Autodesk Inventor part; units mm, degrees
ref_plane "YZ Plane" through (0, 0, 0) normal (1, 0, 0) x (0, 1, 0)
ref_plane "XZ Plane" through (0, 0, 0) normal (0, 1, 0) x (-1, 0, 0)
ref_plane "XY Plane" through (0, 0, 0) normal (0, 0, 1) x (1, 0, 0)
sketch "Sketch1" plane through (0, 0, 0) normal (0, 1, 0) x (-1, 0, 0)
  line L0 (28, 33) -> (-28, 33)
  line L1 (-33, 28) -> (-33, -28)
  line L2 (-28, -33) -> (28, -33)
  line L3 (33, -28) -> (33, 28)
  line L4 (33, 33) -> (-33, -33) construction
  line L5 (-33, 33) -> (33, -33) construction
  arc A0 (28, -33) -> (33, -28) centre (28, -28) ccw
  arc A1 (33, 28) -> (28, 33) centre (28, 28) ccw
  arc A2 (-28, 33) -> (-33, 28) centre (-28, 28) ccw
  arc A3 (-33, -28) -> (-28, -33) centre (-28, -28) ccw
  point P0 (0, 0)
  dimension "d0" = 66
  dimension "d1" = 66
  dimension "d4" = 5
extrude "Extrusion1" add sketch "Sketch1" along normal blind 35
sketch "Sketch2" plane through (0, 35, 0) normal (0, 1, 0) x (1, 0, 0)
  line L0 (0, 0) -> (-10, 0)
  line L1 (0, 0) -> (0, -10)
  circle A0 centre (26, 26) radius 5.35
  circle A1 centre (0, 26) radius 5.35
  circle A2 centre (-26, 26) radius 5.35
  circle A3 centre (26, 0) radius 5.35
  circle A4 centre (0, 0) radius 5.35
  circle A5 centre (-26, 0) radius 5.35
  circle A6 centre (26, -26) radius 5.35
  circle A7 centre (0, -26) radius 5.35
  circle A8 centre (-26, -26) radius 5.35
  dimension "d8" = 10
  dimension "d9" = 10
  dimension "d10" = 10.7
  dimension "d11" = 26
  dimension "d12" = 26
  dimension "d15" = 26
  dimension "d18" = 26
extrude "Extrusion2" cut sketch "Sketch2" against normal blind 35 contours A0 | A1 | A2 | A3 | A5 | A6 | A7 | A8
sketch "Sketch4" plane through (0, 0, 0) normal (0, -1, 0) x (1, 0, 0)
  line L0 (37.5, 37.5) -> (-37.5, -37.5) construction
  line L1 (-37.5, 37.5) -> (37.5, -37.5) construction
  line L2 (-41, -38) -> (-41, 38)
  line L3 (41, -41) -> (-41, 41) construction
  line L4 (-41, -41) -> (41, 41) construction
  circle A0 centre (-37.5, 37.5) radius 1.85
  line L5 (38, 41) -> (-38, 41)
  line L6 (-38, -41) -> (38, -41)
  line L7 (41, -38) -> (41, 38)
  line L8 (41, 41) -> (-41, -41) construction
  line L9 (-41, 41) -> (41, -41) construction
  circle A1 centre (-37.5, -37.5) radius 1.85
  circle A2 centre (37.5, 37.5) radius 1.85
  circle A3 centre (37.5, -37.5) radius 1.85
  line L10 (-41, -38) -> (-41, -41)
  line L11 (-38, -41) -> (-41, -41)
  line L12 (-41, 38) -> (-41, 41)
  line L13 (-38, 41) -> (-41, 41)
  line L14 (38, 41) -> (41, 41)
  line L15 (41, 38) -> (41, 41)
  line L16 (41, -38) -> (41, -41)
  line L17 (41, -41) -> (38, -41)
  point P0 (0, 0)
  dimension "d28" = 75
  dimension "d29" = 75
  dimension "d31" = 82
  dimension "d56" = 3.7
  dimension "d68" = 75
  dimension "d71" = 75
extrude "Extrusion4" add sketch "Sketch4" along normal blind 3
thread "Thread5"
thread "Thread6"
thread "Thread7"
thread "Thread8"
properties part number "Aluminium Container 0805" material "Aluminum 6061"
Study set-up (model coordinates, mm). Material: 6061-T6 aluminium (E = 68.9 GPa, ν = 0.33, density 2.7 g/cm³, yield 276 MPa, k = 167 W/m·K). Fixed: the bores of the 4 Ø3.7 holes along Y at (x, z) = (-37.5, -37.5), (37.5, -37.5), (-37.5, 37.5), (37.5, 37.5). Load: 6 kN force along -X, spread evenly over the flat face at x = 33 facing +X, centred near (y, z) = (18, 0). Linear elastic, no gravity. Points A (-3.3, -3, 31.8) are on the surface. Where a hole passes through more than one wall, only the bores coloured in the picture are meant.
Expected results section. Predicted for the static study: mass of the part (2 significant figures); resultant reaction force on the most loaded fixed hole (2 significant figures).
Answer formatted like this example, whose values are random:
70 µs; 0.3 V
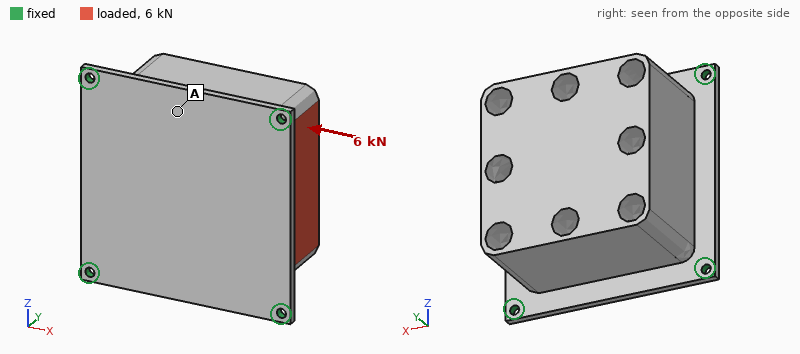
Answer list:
400 g; 1.9 kN
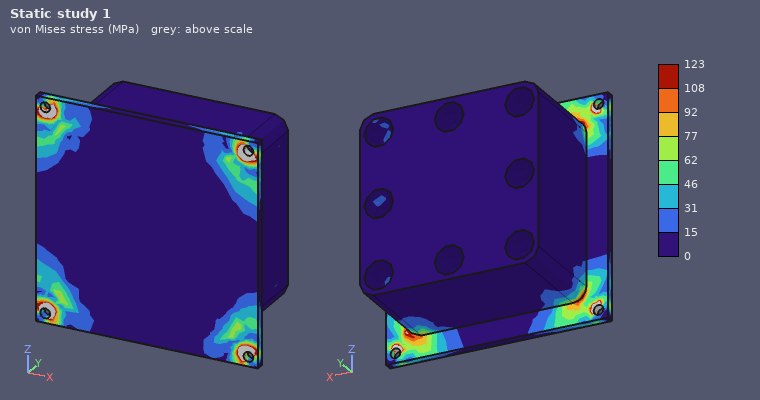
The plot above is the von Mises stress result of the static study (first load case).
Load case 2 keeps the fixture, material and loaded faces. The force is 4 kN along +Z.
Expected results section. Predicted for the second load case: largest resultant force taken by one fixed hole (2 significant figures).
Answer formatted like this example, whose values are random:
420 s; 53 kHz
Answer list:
1.6 kN
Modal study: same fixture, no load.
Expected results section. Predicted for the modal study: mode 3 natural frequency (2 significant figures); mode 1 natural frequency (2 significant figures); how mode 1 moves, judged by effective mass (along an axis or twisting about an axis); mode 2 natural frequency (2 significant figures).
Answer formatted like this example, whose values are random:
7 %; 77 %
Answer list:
2500 Hz; 2100 Hz; along Y; 2500 Hz
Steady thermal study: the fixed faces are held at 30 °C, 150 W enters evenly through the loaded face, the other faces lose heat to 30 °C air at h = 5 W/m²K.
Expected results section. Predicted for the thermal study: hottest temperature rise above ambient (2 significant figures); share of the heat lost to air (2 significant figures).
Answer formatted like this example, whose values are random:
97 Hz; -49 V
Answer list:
80 K; 6.1 %
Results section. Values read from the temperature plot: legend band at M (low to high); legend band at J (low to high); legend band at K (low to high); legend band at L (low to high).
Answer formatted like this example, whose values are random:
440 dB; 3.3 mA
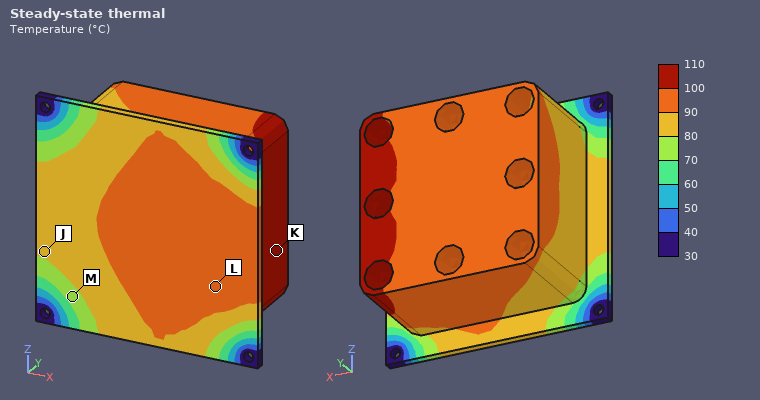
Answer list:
70 to 80 °C; 80 to 90 °C; 100 to 110 °C; 90 to 100 °C
